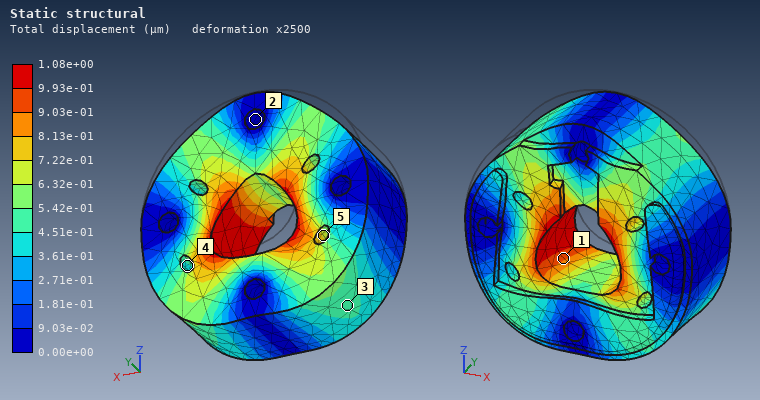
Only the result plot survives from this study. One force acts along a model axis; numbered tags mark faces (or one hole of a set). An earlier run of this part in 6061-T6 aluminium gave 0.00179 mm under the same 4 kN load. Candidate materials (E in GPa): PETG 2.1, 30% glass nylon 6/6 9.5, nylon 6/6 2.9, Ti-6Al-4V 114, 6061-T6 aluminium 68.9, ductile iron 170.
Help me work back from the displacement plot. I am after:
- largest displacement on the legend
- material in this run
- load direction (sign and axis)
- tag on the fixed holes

1.08e+00 µm
Ti-6Al-4V
-Z
2
